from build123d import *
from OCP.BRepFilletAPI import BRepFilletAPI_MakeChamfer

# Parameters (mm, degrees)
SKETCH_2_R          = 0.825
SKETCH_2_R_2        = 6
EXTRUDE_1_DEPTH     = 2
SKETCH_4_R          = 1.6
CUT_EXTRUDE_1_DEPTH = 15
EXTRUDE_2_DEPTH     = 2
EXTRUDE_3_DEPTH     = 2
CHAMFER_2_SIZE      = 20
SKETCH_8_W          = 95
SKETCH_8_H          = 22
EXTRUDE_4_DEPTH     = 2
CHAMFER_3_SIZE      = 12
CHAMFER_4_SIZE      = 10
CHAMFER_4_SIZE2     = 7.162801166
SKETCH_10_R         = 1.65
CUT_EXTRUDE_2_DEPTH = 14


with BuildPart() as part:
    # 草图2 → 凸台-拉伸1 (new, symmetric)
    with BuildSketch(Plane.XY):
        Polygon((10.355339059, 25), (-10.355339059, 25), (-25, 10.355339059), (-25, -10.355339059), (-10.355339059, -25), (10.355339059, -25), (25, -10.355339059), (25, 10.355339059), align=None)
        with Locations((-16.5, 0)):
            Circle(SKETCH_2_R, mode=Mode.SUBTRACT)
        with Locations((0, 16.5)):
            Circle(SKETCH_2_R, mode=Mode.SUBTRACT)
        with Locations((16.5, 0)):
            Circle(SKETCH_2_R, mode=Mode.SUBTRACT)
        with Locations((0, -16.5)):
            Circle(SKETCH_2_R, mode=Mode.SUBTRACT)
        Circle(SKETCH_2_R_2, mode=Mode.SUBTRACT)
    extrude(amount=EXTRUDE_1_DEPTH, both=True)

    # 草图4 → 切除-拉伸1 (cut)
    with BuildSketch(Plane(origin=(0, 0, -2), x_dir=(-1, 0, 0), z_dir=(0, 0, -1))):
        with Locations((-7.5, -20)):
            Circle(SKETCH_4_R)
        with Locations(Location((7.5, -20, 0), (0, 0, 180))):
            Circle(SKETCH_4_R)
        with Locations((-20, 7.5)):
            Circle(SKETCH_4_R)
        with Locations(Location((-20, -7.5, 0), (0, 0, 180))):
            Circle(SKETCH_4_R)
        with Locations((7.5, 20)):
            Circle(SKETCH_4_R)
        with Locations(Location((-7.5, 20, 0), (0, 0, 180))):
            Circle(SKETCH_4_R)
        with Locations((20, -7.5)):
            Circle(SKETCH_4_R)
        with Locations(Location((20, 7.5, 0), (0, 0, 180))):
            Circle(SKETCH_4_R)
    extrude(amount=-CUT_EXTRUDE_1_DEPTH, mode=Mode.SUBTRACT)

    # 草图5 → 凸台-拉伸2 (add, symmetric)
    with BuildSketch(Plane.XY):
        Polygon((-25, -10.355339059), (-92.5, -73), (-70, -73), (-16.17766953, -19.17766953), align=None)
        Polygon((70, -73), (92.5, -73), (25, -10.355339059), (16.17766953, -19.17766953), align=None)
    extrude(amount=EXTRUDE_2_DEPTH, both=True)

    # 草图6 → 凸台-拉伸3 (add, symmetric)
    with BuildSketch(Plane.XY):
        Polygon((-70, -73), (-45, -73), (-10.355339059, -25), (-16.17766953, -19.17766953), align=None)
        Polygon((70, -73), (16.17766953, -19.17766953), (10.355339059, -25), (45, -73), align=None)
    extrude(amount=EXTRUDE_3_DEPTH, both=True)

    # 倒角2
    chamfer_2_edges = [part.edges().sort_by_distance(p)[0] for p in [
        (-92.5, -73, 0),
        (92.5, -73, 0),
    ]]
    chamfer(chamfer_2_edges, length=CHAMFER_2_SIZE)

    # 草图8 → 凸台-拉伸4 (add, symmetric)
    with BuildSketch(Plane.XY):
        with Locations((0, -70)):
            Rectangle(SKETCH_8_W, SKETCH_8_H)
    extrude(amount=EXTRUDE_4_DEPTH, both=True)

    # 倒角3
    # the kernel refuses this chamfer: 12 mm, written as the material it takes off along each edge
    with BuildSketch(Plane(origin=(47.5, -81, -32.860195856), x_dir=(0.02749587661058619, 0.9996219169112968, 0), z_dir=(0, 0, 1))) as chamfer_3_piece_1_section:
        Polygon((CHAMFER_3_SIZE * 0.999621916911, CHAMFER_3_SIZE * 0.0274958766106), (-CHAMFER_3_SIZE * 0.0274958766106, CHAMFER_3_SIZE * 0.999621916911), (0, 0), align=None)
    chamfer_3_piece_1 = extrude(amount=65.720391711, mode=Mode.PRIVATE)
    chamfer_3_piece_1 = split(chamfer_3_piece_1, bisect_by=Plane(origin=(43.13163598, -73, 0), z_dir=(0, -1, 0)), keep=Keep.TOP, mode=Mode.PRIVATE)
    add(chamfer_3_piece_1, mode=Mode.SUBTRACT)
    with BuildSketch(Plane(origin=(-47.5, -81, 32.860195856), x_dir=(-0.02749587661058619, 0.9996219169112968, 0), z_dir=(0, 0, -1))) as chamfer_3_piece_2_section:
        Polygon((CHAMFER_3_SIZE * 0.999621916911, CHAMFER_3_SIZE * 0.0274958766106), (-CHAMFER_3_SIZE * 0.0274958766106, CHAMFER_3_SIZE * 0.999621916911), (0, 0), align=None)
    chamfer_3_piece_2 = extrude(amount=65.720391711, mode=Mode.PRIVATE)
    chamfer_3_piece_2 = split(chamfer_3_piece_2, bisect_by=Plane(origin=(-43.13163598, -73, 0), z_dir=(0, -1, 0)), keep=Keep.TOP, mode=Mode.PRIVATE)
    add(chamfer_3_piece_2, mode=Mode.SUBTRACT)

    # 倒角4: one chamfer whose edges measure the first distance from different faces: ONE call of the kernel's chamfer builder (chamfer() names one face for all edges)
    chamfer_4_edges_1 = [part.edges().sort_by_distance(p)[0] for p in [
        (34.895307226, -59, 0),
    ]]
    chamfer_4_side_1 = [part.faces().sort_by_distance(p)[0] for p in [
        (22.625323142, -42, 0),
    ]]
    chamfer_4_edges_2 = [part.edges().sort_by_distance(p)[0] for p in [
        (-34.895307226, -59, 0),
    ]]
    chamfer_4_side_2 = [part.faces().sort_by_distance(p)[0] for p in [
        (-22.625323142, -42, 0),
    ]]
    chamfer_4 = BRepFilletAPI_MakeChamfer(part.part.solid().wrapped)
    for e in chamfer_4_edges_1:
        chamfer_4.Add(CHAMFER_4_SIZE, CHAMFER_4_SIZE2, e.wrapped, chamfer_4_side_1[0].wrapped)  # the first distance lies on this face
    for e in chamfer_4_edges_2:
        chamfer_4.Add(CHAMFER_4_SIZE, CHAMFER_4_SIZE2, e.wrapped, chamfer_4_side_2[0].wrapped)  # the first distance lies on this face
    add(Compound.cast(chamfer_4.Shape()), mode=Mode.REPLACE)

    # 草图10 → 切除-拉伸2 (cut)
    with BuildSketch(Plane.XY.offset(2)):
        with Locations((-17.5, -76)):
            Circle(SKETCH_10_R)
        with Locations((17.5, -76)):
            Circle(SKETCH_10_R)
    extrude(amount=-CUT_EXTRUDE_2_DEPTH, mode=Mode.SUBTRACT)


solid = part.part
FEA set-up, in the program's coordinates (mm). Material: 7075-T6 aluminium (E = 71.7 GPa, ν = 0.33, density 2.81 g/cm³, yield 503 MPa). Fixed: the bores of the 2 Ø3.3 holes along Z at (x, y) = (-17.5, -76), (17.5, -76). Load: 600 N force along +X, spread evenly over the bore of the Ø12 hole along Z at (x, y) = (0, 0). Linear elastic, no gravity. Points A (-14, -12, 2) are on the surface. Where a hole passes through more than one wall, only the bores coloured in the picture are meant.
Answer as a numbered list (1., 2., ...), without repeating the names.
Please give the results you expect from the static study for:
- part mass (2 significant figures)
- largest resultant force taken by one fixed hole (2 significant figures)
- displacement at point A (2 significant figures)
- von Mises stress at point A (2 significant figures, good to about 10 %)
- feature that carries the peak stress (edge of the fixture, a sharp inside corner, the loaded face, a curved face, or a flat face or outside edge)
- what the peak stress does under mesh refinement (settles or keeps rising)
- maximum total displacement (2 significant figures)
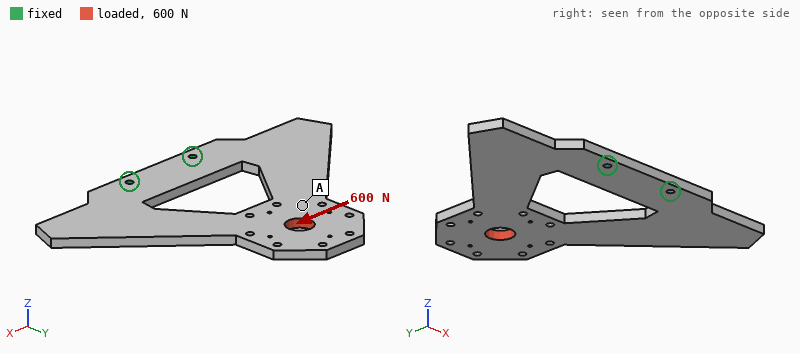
1. 85 g
2. 1.2 kN
3. 0.075 mm
4. 7.0 MPa
5. edge of the fixture
6. keeps rising
7. 0.10 mm
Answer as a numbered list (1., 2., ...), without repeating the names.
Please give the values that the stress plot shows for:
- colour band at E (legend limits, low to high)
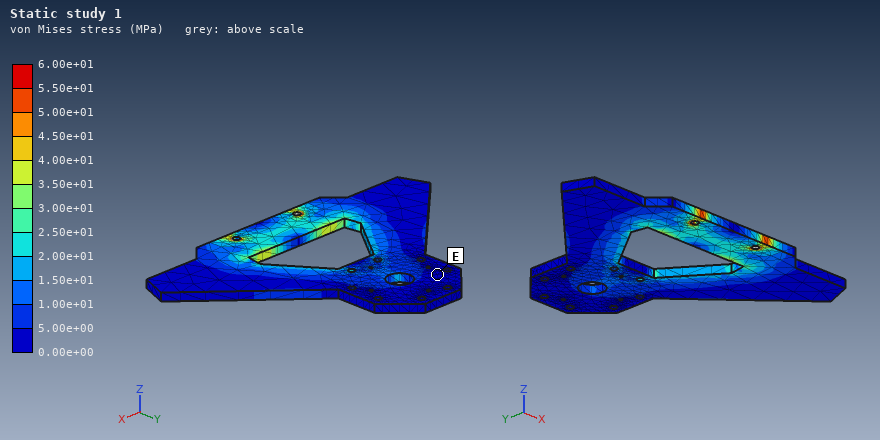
1. 0.00e+00 to 5.00e+00 MPa
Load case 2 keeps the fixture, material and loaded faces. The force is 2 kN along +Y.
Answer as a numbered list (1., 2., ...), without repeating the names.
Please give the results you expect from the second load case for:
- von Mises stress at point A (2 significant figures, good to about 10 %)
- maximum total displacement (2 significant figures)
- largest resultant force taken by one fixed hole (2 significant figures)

1. 12 MPa
2. 45 µm
3. 1.1 kN
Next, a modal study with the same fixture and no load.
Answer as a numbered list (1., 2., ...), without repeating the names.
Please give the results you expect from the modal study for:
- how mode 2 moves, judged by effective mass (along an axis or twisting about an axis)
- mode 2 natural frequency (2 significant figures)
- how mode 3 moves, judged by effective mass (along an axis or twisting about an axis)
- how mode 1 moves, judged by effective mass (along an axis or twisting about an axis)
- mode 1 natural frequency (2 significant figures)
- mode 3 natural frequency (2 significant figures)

1. twisting about Y
2. 710 Hz
3. along Z
4. along Z
5. 310 Hz
6. 970 Hz
